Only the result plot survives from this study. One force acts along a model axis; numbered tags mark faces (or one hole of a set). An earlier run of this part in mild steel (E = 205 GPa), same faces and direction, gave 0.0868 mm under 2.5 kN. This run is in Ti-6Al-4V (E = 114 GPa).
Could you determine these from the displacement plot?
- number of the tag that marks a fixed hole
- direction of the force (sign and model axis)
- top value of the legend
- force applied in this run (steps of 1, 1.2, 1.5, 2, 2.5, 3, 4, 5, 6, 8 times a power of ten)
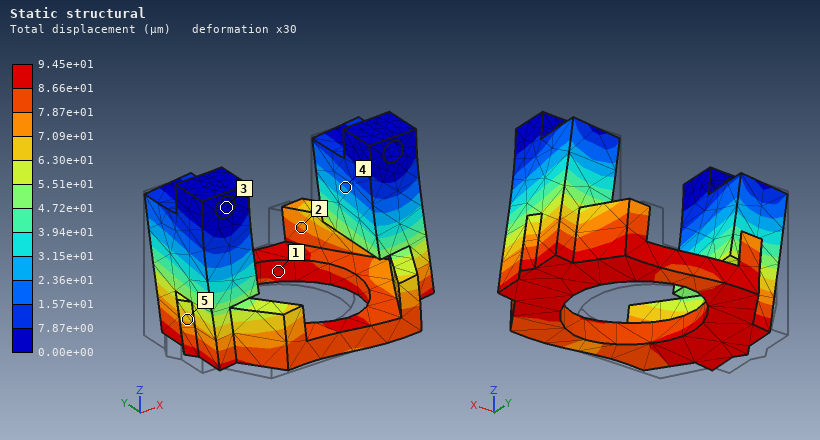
3
+X
9.45e+01 µm
1.5 kN
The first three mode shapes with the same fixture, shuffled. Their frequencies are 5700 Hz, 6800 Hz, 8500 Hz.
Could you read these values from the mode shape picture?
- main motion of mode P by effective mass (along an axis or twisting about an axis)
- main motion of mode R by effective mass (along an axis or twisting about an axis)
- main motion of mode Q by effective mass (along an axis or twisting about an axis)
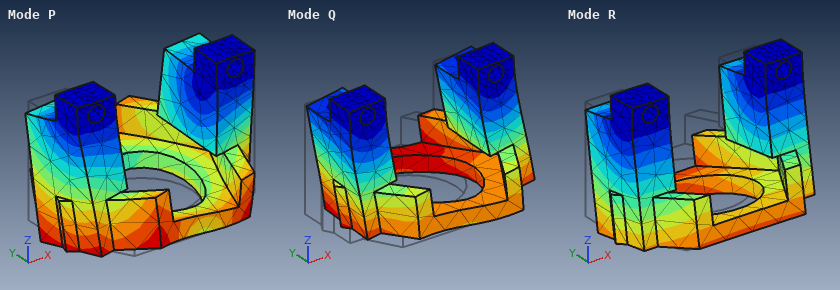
twisting about Z
along Y
along X
